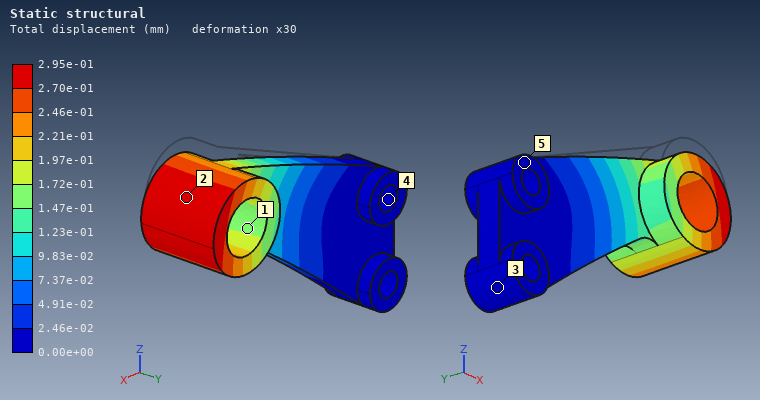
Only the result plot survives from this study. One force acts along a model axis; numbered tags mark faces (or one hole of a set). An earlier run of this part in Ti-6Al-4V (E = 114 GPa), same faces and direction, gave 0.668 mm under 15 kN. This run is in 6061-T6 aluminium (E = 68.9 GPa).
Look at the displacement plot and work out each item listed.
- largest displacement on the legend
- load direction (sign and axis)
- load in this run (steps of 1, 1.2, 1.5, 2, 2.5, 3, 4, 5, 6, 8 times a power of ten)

2.95e-01 mm
-Z
4 kN
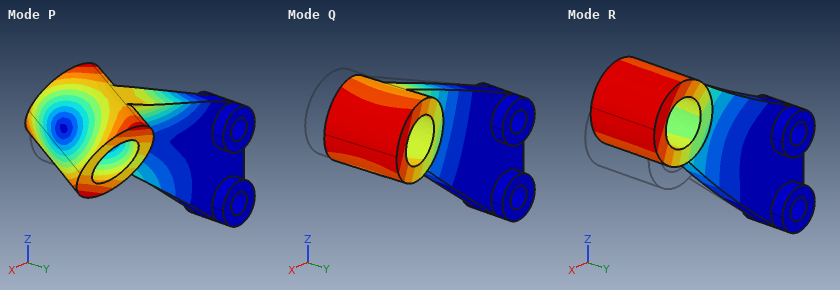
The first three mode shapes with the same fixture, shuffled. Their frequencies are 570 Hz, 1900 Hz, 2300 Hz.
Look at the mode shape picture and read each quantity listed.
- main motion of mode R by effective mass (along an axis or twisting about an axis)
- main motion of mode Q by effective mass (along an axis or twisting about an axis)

along Z
along Y
